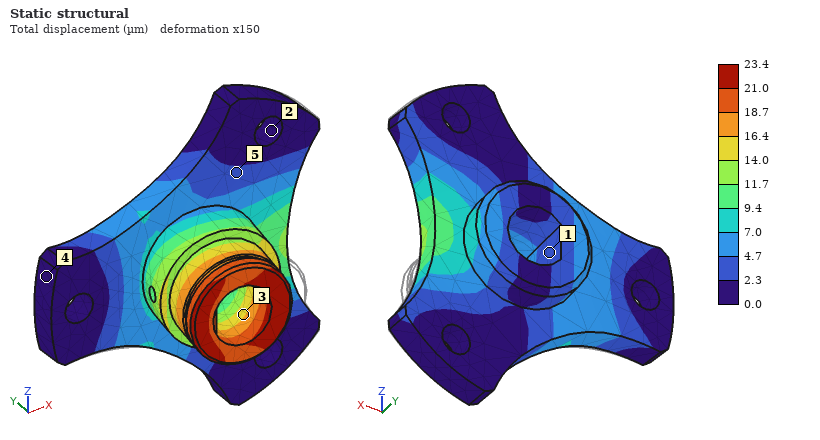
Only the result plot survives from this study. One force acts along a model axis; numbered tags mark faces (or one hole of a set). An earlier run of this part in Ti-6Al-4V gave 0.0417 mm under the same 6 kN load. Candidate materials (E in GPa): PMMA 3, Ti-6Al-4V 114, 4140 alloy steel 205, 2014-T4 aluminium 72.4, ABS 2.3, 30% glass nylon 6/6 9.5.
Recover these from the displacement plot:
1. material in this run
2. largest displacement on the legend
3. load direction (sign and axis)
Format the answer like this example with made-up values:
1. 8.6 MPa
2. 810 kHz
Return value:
1. 4140 alloy steel
2. 23.4 µm
3. -X
